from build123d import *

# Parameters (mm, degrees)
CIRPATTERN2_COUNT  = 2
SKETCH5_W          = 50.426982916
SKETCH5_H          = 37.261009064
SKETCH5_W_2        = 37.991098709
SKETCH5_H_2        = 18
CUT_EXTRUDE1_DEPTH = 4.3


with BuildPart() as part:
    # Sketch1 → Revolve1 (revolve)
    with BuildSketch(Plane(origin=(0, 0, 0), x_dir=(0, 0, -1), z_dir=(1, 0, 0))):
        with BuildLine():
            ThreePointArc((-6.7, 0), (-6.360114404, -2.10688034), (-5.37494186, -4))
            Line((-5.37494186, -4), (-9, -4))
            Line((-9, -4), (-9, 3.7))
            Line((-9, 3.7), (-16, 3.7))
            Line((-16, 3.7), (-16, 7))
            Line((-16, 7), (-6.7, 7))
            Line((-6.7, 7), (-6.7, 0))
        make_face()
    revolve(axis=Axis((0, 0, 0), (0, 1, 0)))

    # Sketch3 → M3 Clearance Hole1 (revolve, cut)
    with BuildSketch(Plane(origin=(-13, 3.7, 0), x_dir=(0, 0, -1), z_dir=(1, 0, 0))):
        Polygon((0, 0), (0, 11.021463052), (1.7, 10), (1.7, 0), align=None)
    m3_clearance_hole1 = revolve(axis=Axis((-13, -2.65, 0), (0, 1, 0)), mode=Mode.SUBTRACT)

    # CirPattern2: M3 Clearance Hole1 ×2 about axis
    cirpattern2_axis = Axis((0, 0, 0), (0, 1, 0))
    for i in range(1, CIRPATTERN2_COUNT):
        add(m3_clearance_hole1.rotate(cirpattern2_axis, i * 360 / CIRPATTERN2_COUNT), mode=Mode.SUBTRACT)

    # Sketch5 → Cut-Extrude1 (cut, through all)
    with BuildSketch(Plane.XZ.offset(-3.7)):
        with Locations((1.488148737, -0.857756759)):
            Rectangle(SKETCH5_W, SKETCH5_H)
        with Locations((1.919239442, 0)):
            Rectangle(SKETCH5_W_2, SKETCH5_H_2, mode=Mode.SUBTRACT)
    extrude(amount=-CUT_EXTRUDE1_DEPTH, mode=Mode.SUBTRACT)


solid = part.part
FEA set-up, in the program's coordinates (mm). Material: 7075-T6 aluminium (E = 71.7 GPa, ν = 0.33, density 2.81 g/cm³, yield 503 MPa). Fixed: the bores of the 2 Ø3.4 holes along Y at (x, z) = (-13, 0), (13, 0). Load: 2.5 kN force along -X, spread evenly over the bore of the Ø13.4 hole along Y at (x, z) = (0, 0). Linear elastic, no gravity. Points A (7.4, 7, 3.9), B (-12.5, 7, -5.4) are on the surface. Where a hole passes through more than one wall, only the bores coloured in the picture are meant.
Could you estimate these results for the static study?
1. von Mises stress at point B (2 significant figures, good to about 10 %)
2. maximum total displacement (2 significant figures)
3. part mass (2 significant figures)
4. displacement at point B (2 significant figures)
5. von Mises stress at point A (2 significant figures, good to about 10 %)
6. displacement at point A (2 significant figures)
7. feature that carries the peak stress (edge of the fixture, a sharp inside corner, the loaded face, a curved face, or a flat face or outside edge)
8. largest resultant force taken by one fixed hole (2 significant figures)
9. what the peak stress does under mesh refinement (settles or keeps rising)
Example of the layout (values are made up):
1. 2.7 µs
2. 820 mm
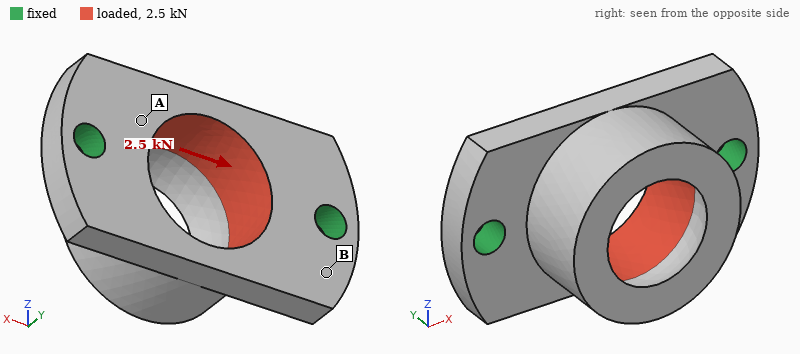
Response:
1. 11 MPa
2. 7.7 µm
3. 6.2 g
4. 3.6 µm
5. 29 MPa
6. 3.6 µm
7. edge of the fixture
8. 1.3 kN
9. keeps rising
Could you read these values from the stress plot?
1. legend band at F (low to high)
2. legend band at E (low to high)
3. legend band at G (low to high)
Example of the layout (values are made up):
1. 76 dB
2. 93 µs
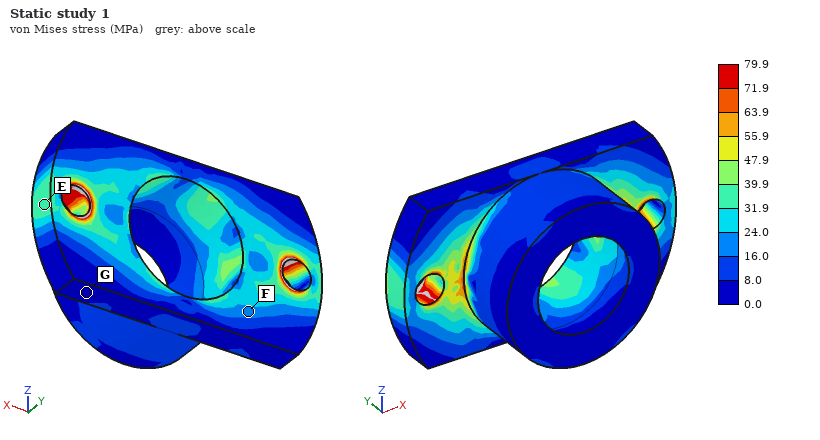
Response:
1. 16.0 to 24.0 MPa
2. 31.9 to 39.9 MPa
3. 0.0 to 8.0 MPa
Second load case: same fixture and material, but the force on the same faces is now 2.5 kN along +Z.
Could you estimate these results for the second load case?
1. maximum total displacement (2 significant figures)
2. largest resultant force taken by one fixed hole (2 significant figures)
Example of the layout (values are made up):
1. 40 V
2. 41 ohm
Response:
1. 42 µm
2. 1.3 kN
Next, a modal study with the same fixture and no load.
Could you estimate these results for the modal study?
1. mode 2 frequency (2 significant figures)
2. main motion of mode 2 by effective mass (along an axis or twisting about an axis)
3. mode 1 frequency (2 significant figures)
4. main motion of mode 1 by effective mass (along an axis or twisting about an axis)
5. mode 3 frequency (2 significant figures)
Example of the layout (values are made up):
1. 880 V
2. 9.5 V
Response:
1. 23 kHz
2. along Y
3. 13 kHz
4. along Z
5. 34 kHz
